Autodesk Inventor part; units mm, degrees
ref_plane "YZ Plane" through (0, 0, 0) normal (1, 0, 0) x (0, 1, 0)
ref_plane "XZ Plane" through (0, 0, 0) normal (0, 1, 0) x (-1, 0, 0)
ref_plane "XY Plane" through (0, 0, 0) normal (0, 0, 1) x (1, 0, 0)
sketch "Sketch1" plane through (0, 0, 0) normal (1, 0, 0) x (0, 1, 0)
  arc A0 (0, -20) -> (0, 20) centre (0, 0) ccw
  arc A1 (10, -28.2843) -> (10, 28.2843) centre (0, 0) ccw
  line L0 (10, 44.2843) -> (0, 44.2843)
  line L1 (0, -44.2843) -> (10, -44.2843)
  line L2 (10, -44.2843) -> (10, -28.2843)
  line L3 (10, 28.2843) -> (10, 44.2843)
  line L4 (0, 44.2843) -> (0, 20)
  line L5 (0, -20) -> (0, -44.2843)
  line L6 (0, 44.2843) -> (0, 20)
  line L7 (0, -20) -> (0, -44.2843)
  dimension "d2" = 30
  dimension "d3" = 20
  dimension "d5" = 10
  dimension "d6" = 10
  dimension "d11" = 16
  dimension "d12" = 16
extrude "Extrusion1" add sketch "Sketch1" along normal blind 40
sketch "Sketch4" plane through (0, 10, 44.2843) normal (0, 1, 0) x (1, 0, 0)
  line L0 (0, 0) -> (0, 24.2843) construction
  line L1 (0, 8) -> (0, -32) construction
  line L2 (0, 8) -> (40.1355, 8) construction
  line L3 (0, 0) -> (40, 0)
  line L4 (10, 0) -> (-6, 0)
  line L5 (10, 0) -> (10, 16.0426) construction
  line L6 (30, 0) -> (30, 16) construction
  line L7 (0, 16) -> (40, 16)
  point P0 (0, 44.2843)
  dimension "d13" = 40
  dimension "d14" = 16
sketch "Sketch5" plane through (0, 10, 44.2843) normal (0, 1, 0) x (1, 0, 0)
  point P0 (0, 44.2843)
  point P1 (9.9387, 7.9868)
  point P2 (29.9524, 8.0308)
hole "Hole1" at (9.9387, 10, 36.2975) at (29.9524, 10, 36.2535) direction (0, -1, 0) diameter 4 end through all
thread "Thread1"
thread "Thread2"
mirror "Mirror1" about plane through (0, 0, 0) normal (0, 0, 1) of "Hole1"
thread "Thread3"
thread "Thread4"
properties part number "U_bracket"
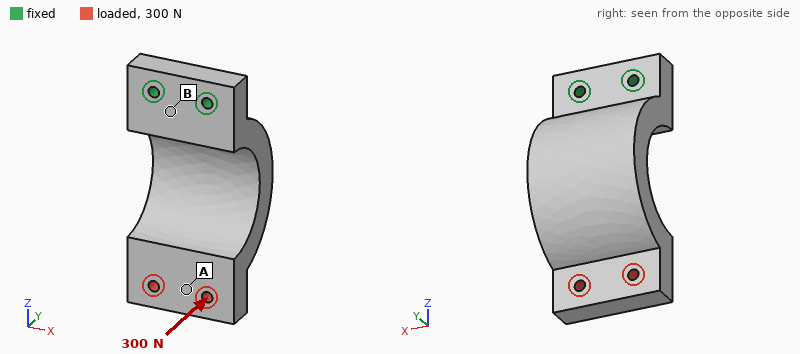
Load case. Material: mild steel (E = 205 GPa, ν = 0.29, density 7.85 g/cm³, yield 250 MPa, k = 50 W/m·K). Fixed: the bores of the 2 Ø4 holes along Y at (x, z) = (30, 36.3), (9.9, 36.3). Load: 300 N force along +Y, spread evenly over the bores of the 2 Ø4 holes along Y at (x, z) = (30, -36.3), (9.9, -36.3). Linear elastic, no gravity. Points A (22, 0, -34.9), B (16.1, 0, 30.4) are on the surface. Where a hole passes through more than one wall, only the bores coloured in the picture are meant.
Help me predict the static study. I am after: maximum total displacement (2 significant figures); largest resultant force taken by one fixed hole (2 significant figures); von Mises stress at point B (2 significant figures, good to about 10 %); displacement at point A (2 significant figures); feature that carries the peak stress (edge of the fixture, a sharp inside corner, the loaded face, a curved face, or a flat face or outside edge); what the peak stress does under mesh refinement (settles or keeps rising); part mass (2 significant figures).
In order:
85 µm
160 N
23 MPa
72 µm
edge of the fixture
keeps rising
340 g
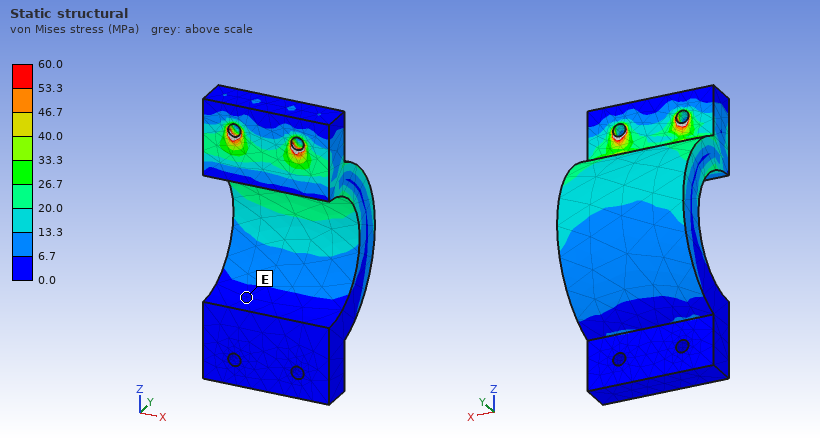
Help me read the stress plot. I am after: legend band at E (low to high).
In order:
0.0 to 6.7 MPa
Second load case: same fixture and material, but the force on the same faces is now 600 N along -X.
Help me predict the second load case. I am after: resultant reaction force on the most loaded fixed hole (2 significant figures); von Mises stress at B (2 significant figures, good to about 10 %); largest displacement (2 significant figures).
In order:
1.9 kN
20 MPa
53 µm
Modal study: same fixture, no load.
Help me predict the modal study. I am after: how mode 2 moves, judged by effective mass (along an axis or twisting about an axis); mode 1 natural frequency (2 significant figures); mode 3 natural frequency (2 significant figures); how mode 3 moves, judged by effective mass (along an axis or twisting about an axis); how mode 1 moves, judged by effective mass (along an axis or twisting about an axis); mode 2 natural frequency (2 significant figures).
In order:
along X
1000 Hz
3500 Hz
along Z
along Y
1900 Hz
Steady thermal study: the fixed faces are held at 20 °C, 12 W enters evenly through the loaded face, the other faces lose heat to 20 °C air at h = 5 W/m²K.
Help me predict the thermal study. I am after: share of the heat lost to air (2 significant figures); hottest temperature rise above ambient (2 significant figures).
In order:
12 %
50 K
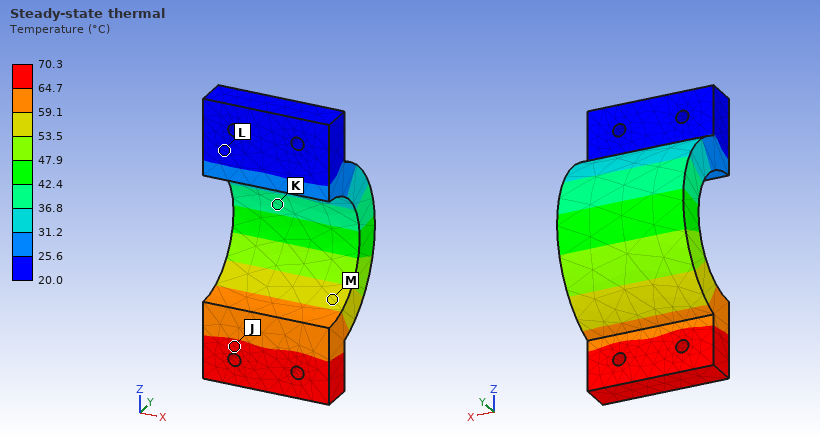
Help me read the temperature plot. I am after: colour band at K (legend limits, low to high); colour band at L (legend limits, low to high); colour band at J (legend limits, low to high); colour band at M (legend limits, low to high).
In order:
36.8 to 42.4 °C
20.0 to 25.6 °C
64.7 to 70.3 °C
53.5 to 59.1 °C
